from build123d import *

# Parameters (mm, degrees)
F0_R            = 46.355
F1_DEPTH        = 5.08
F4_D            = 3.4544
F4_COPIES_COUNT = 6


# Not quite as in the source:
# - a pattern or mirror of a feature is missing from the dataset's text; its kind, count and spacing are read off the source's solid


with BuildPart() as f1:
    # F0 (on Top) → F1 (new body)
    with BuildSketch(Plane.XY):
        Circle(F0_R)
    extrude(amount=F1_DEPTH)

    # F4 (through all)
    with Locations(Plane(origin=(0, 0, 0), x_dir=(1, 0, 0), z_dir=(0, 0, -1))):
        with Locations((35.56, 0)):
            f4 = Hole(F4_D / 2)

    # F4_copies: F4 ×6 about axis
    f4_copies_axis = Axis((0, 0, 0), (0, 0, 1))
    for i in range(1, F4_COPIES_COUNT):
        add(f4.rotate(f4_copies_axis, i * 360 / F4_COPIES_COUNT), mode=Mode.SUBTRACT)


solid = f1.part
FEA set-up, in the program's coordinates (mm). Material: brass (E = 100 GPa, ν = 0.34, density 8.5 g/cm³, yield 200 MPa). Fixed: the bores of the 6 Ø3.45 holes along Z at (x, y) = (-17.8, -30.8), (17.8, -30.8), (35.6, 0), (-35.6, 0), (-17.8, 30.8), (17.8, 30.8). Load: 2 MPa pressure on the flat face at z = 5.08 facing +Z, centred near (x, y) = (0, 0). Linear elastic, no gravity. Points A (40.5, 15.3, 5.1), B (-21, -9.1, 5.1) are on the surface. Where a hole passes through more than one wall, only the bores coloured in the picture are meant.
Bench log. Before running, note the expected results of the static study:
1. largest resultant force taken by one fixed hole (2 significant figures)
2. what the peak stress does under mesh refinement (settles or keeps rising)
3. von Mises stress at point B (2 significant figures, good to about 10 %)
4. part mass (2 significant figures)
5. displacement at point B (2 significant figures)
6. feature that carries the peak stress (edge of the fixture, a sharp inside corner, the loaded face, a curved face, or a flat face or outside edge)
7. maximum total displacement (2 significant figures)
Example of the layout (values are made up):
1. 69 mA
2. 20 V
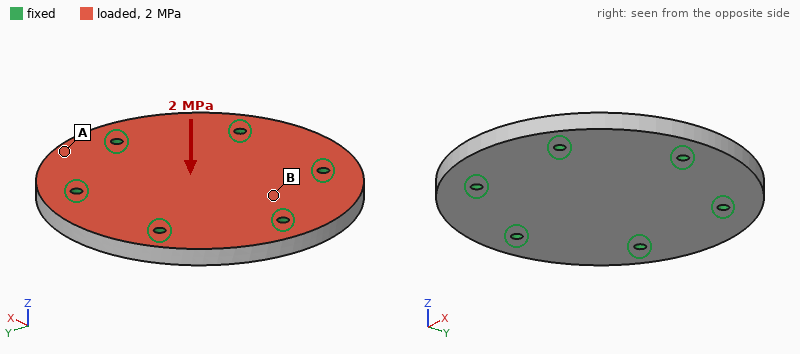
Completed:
1. 2.2 kN
2. keeps rising
3. 35 MPa
4. 290 g
5. 28 µm
6. edge of the fixture
7. 57 µm
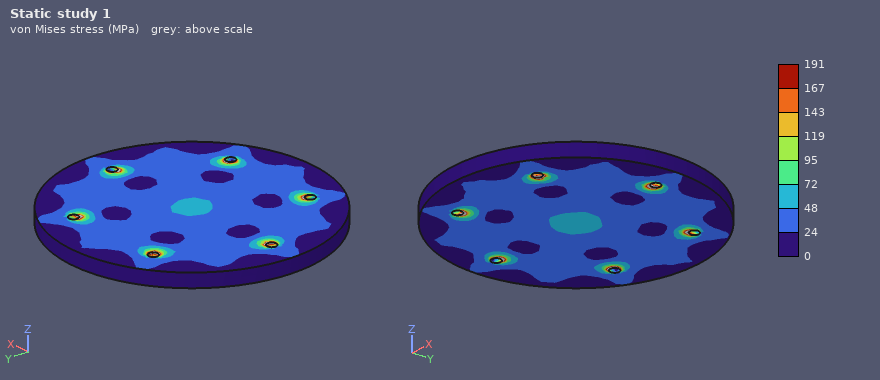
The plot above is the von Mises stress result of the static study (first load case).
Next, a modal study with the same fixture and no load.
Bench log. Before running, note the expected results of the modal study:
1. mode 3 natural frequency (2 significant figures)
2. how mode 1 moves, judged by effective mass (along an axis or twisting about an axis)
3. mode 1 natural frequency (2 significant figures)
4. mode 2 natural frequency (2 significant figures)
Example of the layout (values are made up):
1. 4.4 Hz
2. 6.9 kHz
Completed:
1. 8500 Hz
2. along Z
3. 5300 Hz
4. 8000 Hz
